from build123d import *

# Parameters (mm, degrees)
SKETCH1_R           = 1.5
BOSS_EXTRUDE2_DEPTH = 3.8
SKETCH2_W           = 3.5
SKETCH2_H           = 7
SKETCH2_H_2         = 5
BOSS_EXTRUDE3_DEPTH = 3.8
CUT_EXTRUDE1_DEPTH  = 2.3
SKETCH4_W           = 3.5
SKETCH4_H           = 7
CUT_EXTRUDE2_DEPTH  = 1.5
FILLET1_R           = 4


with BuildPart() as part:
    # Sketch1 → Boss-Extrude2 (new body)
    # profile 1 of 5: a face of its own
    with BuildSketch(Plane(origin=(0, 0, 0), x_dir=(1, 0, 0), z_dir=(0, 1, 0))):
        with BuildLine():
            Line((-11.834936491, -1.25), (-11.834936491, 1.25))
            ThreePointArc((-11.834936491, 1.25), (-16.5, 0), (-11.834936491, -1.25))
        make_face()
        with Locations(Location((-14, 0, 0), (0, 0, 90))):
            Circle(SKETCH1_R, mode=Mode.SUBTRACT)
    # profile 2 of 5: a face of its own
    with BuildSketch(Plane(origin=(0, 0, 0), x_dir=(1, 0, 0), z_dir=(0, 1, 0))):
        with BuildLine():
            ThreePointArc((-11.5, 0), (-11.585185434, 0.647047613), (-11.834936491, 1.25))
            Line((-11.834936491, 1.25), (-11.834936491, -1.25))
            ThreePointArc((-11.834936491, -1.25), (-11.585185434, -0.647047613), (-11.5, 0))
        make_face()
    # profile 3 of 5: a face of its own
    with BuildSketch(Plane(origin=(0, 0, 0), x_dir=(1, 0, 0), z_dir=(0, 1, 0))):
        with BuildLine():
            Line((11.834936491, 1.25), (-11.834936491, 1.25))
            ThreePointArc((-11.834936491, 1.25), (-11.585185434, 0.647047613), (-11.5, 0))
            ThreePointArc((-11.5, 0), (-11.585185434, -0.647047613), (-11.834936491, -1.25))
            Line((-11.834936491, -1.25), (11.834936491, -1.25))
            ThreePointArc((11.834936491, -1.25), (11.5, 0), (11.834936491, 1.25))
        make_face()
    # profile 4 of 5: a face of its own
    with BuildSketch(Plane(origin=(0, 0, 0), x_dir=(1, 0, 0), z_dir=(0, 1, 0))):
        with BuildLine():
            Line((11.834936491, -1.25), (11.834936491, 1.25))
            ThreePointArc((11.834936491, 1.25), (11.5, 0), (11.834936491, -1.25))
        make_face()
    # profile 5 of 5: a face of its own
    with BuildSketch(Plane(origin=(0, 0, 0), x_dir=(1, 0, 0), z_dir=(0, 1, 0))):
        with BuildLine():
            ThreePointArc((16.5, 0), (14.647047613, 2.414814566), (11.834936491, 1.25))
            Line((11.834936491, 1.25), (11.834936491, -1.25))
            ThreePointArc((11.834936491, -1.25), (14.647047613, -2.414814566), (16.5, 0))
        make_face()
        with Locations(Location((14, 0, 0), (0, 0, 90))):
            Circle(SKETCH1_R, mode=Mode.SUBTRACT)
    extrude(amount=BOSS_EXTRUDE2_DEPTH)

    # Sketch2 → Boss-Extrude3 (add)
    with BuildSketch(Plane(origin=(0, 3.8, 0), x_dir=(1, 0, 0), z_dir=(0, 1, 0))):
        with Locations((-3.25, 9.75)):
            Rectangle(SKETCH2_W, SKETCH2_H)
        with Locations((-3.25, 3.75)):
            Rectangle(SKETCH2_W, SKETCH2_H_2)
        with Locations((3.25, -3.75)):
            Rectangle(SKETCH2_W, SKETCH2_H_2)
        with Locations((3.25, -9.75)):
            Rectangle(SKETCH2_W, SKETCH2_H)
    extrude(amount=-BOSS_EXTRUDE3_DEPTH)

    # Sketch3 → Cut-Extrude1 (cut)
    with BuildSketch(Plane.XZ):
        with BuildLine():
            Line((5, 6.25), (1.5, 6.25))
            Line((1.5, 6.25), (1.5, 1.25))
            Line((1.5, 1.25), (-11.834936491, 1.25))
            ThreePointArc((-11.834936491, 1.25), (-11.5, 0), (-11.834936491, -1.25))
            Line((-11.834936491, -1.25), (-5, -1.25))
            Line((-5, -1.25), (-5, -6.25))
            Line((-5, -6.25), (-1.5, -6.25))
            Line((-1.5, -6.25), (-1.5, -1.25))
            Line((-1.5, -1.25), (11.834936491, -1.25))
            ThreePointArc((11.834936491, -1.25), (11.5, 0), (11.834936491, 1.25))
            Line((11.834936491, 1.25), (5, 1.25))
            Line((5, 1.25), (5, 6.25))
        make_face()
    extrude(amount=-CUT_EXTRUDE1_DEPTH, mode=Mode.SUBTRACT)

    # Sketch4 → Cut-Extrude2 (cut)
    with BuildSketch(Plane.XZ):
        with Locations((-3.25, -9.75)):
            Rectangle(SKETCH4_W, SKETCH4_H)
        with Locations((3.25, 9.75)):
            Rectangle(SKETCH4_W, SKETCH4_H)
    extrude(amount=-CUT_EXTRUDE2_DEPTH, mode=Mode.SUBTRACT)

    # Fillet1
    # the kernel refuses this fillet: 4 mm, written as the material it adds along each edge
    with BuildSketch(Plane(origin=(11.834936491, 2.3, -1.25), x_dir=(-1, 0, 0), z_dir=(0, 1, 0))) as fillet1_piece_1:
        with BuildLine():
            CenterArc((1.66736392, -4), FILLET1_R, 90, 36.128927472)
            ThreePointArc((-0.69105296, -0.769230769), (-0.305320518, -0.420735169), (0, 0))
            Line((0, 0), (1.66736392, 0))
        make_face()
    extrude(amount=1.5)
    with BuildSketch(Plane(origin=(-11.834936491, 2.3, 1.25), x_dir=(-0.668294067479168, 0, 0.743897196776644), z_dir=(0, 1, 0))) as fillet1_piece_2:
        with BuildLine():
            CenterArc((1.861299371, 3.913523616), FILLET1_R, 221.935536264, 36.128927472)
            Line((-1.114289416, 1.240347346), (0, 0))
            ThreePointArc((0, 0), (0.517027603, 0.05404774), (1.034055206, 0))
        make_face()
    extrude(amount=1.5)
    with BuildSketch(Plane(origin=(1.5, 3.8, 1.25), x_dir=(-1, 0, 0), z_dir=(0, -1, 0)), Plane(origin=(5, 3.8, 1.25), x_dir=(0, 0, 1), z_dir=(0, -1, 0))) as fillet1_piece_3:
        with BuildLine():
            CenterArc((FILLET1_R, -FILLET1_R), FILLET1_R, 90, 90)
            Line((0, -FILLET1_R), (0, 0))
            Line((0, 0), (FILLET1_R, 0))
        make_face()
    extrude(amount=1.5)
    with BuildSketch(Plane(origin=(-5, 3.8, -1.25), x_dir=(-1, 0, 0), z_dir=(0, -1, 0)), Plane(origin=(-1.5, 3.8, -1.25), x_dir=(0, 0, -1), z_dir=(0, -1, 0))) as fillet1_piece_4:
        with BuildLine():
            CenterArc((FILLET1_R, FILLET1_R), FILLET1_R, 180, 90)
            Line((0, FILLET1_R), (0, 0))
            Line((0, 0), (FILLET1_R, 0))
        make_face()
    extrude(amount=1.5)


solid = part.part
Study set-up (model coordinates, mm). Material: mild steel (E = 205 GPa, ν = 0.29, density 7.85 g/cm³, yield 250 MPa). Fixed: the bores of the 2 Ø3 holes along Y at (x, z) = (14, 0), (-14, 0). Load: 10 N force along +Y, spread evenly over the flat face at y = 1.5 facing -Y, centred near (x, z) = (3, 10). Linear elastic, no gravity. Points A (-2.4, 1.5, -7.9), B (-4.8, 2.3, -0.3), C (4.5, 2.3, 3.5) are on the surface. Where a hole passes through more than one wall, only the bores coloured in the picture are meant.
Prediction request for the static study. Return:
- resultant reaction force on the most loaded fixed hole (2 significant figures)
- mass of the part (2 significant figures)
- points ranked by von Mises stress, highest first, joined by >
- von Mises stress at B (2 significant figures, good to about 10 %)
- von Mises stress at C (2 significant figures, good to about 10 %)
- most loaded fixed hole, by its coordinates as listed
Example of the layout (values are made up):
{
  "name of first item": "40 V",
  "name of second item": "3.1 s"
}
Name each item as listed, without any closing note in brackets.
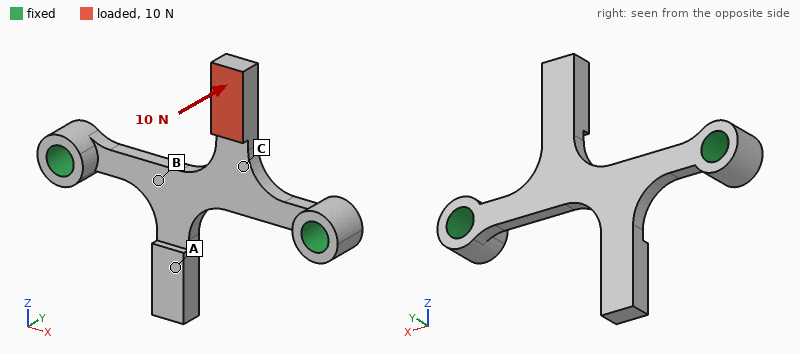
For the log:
{
  "resultant reaction force on the most loaded fixed hole": "7.1 N",
  "mass of the part": "2.9 g",
  "points ranked by von Mises stress, highest first, joined by >": "C > B > A",
  "von Mises stress at B": "28 MPa",
  "von Mises stress at C": "46 MPa",
  "most loaded fixed hole, by its coordinates as listed": "(14, 0)"
}
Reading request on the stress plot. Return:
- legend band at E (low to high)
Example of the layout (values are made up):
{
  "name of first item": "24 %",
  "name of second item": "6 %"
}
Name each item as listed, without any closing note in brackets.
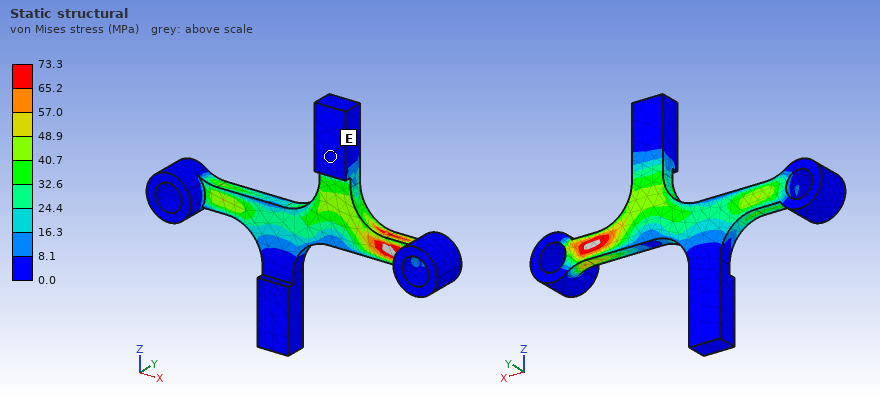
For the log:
{
  "legend band at E": "0.0 to 8.1 MPa"
}
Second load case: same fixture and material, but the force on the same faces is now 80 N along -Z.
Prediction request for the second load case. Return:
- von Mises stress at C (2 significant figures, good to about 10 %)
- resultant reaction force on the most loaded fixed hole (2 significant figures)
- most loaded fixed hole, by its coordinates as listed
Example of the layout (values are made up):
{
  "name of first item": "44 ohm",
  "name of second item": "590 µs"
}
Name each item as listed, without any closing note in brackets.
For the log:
{
  "von Mises stress at C": "91 MPa",
  "resultant reaction force on the most loaded fixed hole": "55 N",
  "most loaded fixed hole, by its coordinates as listed": "(14, 0)"
}
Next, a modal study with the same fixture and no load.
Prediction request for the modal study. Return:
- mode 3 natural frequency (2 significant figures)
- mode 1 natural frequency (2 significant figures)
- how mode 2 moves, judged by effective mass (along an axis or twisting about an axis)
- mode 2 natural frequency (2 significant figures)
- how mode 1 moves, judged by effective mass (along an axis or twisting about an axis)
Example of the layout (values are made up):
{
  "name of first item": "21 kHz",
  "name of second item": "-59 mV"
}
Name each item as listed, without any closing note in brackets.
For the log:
{
  "mode 3 natural frequency": "11 kHz",
  "mode 1 natural frequency": "3100 Hz",
  "how mode 2 moves, judged by effective mass": "along Y",
  "mode 2 natural frequency": "4700 Hz",
  "how mode 1 moves, judged by effective mass": "twisting about X"
}
